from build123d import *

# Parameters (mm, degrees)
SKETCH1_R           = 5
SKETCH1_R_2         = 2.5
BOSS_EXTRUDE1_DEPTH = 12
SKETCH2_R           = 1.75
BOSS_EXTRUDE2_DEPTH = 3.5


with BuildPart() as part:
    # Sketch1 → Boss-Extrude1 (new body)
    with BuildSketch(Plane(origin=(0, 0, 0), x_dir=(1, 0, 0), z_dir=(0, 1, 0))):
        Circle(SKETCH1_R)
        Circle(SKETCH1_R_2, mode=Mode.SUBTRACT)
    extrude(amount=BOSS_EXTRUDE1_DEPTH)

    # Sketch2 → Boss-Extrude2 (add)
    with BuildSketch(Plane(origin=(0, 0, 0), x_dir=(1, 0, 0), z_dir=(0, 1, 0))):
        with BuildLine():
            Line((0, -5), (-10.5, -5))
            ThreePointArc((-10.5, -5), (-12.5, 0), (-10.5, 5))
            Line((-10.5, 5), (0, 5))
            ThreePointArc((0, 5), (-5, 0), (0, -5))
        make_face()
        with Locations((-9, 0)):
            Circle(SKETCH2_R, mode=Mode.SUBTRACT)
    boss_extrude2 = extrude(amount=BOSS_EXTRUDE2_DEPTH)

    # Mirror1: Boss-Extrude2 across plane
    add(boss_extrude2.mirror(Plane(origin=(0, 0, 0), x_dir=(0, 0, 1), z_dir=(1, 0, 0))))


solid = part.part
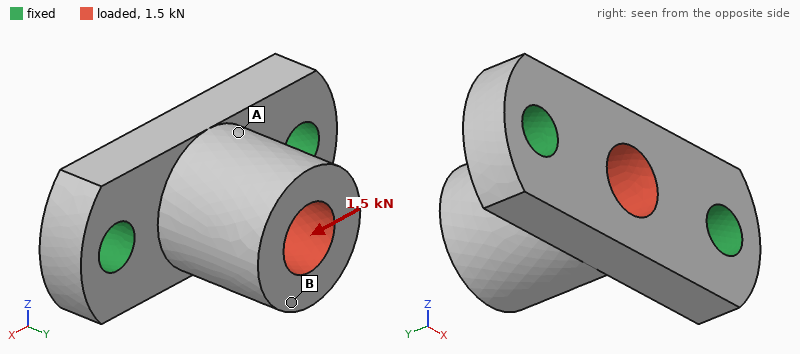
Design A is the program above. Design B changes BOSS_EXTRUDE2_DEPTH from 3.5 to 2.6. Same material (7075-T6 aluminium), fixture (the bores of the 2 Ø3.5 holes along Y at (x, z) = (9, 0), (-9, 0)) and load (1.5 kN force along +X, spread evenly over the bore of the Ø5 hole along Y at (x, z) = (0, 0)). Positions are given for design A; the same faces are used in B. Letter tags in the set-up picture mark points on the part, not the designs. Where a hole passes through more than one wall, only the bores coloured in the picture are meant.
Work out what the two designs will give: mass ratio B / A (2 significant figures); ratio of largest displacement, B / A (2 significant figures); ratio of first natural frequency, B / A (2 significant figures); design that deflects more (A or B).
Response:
0.89
1.6
0.72
B
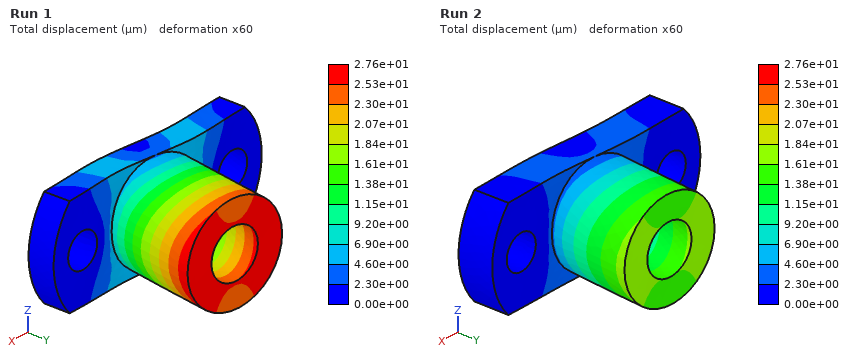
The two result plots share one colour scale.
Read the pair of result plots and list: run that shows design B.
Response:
Run 1
